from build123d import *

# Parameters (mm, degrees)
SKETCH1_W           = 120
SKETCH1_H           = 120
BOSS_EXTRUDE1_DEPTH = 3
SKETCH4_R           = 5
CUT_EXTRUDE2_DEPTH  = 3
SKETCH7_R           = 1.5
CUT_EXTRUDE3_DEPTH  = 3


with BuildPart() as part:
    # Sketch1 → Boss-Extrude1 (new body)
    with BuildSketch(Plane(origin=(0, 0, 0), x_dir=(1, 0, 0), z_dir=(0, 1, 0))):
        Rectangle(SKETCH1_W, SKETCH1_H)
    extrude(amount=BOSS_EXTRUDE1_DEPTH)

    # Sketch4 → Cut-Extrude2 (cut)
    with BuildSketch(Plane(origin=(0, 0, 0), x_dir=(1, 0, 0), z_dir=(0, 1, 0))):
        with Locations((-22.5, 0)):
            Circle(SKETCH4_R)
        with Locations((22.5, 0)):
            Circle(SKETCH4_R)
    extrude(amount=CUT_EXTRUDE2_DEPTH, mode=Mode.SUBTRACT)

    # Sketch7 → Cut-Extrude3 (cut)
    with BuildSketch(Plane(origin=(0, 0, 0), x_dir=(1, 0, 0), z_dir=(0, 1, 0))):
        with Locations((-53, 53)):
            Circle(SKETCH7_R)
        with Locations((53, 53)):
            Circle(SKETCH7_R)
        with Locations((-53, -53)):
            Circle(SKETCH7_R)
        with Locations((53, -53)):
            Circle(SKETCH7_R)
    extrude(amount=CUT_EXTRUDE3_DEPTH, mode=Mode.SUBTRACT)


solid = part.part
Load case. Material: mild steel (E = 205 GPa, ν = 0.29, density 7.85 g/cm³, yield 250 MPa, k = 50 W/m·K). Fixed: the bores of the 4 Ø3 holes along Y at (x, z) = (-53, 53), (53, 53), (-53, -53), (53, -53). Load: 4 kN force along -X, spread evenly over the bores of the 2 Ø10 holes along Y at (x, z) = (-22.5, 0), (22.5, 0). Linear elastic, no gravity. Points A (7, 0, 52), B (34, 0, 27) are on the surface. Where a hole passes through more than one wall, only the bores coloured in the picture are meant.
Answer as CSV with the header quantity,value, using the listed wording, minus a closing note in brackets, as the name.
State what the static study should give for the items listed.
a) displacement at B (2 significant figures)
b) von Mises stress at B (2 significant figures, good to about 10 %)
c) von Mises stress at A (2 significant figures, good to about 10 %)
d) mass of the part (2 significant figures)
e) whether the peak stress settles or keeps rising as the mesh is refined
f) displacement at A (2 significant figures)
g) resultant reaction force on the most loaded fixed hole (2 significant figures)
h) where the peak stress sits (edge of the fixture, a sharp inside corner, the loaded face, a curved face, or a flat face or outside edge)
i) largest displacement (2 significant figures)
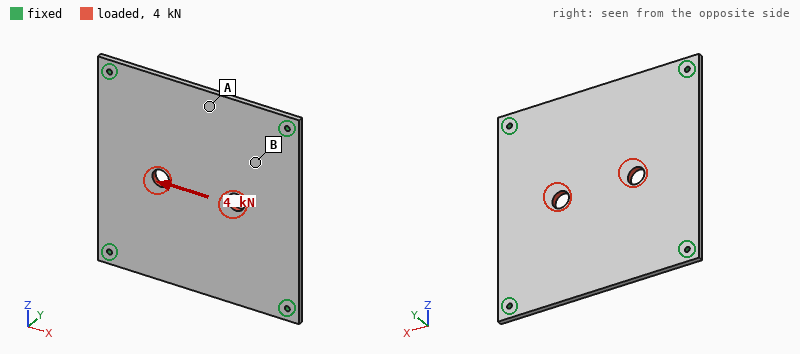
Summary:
quantity,value
displacement at B,4.0 µm
von Mises stress at B,11 MPa
von Mises stress at A,4.8 MPa
mass of the part,330 g
whether the peak stress settles or keeps rising as the mesh is refined,keeps rising
displacement at A,2.6 µm
resultant reaction force on the most loaded fixed hole,1.1 kN
where the peak stress sits,edge of the fixture
largest displacement,6.6 µm
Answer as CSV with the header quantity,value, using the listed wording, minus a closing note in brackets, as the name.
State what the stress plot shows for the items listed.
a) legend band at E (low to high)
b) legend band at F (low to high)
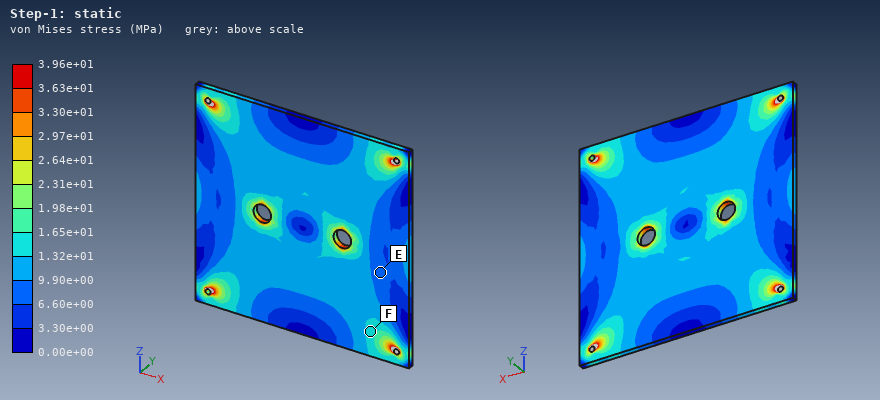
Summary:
quantity,value
legend band at E,6.60e+00 to 9.90e+00 MPa
legend band at F,1.32e+01 to 1.65e+01 MPa
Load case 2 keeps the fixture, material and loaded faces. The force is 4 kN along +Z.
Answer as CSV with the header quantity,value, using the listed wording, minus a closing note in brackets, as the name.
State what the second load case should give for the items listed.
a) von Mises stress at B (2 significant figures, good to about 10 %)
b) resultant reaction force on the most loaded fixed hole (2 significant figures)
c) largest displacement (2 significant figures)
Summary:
quantity,value
von Mises stress at B,12 MPa
resultant reaction force on the most loaded fixed hole,1.1 kN
largest displacement,5.6 µm
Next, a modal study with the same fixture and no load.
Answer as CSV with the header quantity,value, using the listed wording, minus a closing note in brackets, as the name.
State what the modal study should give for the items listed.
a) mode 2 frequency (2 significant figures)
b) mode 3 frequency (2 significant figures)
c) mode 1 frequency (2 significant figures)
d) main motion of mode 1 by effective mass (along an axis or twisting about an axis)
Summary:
quantity,value
mode 2 frequency,1500 Hz
mode 3 frequency,1500 Hz
mode 1 frequency,830 Hz
main motion of mode 1 by effective mass,along Y
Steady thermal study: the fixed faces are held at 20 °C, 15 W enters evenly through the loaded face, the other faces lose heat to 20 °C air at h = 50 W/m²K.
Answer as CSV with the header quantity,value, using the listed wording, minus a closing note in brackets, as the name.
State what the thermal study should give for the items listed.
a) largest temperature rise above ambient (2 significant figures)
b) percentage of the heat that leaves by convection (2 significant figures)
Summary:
quantity,value
largest temperature rise above ambient,23 K
percentage of the heat that leaves by convection,76 %
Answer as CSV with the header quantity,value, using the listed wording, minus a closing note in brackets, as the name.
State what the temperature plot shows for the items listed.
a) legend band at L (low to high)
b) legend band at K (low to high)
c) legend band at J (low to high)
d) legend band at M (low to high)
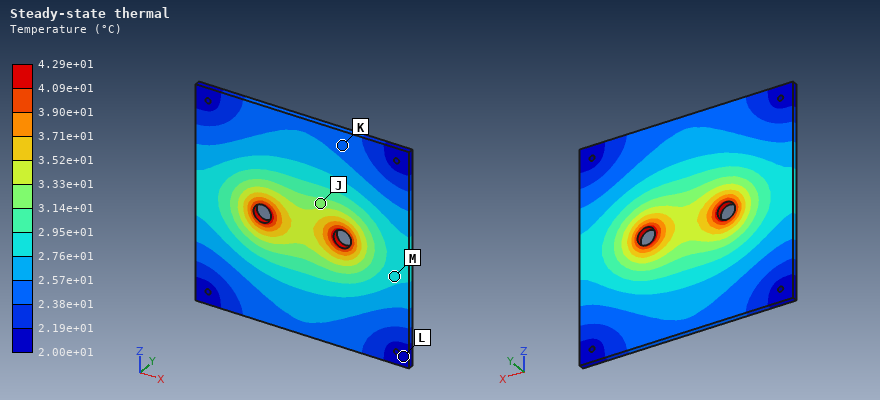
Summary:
quantity,value
legend band at L,2.00e+01 to 2.19e+01 °C
legend band at K,2.38e+01 to 2.57e+01 °C
legend band at J,3.14e+01 to 3.33e+01 °C
legend band at M,2.76e+01 to 2.95e+01 °C
